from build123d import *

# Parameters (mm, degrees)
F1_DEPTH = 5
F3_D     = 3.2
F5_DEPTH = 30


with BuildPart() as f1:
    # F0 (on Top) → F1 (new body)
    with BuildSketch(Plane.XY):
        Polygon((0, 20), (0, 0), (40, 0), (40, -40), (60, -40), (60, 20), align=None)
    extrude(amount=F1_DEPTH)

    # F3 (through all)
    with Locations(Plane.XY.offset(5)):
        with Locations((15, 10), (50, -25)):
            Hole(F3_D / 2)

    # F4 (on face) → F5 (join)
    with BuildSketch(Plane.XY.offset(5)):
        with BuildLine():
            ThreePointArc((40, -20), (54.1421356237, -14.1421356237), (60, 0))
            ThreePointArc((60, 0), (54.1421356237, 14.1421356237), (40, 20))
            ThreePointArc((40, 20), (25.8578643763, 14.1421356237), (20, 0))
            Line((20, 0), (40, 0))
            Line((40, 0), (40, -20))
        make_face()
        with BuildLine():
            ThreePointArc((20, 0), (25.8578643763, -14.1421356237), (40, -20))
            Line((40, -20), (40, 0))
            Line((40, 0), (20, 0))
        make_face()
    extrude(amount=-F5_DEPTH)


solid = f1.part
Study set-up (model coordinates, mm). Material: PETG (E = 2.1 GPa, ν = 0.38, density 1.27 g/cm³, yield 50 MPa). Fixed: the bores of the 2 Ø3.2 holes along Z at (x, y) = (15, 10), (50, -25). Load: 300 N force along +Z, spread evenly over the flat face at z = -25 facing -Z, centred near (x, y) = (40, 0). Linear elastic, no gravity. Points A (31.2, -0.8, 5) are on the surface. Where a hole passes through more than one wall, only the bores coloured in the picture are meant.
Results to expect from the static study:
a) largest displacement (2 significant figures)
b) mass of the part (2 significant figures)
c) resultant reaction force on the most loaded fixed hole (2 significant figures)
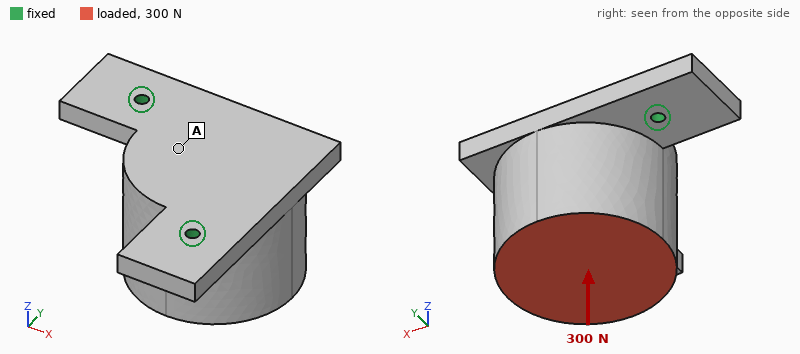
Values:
0.91 mm
54 g
150 N
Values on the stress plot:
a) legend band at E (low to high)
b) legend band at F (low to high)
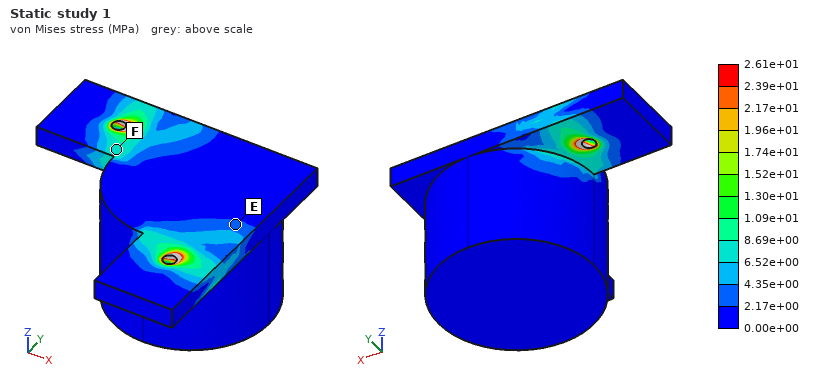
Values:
2.17e+00 to 4.35e+00 MPa
6.52e+00 to 8.69e+00 MPa
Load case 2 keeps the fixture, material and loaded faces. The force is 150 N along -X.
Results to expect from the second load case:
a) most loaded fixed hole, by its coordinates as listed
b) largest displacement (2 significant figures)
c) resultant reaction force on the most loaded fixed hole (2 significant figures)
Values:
(15, 10)
0.97 mm
140 N
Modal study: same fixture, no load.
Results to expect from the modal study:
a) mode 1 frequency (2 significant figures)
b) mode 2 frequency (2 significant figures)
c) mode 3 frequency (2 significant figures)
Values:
390 Hz
1700 Hz
1700 Hz
